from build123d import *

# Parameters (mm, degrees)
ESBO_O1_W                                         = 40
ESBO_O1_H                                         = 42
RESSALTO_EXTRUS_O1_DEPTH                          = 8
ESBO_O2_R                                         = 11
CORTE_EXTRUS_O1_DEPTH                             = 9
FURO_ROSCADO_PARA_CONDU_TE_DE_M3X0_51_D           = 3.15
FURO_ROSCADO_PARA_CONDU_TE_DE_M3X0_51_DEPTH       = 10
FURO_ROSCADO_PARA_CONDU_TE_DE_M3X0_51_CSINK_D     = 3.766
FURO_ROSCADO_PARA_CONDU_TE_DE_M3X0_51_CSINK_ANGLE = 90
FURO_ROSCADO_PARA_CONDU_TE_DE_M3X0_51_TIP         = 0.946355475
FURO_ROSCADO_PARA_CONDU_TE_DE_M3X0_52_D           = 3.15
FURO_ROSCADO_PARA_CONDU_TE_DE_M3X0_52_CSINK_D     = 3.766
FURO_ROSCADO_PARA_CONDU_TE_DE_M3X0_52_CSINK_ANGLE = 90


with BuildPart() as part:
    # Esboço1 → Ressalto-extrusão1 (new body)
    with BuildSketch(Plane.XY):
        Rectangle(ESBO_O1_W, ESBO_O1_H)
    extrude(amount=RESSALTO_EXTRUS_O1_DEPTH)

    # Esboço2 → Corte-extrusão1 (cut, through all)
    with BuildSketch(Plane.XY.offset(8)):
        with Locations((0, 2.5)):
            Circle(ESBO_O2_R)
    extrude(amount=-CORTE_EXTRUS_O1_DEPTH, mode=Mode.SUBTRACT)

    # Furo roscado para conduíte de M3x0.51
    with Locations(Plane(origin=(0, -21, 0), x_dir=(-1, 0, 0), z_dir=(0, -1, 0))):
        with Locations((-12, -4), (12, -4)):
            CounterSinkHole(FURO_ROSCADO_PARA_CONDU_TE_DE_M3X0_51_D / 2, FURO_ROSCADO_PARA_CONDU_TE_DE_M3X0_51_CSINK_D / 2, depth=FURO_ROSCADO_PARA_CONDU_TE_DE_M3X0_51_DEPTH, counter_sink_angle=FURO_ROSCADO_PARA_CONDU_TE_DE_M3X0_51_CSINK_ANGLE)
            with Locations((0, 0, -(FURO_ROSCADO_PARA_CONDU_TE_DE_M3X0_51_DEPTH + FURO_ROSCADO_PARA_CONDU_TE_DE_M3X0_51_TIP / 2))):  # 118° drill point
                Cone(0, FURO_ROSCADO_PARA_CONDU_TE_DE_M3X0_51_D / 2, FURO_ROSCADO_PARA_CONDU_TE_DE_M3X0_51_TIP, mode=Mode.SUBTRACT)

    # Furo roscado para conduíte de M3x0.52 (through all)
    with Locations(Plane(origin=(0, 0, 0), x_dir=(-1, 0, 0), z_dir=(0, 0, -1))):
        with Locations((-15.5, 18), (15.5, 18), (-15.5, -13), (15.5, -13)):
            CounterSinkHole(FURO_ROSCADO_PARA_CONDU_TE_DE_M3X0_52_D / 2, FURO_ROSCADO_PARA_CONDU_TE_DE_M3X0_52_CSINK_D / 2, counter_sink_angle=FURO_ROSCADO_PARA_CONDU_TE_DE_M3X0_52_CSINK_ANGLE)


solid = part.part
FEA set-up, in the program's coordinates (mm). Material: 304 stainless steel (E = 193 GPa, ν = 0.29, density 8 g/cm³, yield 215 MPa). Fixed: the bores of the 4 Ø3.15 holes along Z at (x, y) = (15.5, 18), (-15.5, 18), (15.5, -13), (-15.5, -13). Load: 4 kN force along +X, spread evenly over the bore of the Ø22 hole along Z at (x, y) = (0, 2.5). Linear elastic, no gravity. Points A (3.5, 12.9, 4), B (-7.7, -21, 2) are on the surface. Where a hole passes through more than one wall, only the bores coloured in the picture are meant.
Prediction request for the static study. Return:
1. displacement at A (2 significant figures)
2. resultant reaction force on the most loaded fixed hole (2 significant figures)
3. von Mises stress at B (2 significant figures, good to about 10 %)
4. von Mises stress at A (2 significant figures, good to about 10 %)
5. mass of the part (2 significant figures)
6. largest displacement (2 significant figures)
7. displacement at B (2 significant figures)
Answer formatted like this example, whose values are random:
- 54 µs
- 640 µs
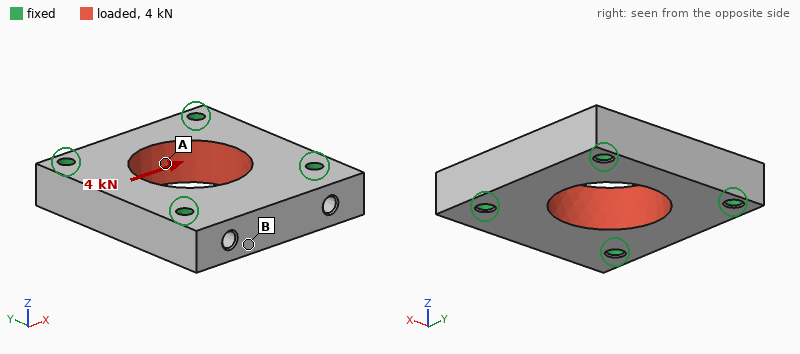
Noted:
- 0.85 µm
- 1.1 kN
- 3.8 MPa
- 16 MPa
- 80 g
- 1.9 µm
- 0.32 µm
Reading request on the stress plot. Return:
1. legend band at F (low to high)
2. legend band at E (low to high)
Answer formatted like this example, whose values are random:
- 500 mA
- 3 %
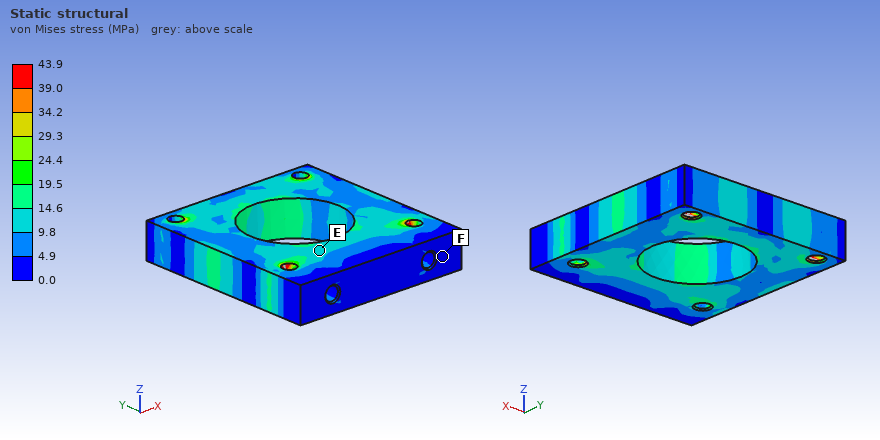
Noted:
- 0.0 to 4.9 MPa
- 9.8 to 14.6 MPa
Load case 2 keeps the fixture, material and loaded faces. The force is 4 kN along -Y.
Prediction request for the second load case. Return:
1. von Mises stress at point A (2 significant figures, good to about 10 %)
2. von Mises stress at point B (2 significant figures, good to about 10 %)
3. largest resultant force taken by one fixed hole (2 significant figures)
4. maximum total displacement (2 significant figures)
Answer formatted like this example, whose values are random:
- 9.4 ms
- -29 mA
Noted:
- 7.4 MPa
- 6.2 MPa
- 1.0 kN
- 2.3 µm
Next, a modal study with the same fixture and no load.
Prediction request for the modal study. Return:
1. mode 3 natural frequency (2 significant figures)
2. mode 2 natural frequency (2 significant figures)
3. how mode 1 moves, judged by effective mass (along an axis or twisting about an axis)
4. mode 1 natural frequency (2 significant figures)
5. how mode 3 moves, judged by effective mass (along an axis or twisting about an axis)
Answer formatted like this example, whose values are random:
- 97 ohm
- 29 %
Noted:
- 29 kHz
- 26 kHz
- along Z
- 25 kHz
- along Z
